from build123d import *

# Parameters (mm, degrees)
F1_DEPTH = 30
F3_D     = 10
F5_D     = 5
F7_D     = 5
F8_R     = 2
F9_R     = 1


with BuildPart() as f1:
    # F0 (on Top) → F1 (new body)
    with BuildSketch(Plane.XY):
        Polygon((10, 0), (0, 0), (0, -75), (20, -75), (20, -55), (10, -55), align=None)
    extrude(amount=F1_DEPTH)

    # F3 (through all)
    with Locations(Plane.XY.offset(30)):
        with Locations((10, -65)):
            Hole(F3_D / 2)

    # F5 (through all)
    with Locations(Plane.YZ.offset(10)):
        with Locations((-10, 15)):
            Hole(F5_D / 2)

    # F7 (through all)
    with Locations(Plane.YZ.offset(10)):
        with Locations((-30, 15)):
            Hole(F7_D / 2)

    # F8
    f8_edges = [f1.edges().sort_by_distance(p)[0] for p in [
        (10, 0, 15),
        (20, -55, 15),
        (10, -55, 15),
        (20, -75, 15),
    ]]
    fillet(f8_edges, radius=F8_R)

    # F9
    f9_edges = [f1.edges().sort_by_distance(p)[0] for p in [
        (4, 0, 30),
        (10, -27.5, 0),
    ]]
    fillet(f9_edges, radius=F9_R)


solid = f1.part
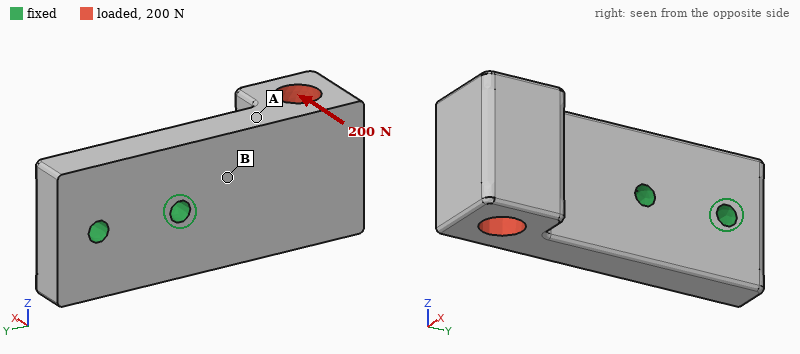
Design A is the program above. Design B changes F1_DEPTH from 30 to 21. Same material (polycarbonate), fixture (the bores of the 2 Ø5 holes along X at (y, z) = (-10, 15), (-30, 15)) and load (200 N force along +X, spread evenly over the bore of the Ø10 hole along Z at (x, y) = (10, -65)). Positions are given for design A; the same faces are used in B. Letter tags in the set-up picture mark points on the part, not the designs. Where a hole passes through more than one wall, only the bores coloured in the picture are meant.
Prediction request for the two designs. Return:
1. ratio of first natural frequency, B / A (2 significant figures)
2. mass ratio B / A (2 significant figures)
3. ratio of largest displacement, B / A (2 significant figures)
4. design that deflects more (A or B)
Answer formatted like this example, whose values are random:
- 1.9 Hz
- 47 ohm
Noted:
- 1.0
- 0.69
- 1.4
- B
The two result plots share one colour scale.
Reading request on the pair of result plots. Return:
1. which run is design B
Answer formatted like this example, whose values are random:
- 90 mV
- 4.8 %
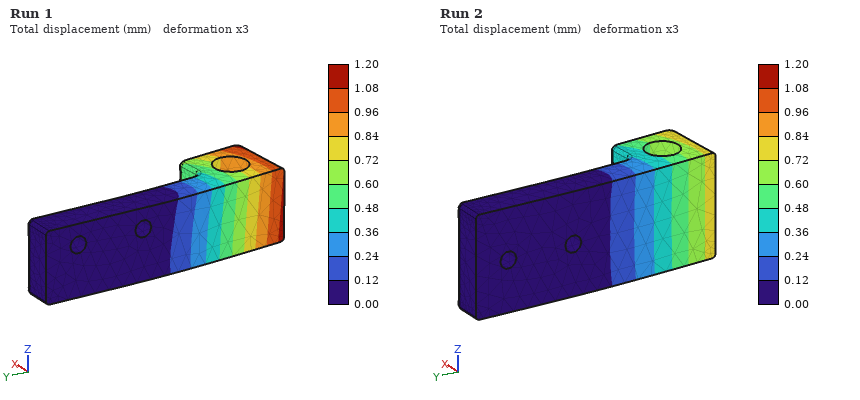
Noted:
- Run 1
